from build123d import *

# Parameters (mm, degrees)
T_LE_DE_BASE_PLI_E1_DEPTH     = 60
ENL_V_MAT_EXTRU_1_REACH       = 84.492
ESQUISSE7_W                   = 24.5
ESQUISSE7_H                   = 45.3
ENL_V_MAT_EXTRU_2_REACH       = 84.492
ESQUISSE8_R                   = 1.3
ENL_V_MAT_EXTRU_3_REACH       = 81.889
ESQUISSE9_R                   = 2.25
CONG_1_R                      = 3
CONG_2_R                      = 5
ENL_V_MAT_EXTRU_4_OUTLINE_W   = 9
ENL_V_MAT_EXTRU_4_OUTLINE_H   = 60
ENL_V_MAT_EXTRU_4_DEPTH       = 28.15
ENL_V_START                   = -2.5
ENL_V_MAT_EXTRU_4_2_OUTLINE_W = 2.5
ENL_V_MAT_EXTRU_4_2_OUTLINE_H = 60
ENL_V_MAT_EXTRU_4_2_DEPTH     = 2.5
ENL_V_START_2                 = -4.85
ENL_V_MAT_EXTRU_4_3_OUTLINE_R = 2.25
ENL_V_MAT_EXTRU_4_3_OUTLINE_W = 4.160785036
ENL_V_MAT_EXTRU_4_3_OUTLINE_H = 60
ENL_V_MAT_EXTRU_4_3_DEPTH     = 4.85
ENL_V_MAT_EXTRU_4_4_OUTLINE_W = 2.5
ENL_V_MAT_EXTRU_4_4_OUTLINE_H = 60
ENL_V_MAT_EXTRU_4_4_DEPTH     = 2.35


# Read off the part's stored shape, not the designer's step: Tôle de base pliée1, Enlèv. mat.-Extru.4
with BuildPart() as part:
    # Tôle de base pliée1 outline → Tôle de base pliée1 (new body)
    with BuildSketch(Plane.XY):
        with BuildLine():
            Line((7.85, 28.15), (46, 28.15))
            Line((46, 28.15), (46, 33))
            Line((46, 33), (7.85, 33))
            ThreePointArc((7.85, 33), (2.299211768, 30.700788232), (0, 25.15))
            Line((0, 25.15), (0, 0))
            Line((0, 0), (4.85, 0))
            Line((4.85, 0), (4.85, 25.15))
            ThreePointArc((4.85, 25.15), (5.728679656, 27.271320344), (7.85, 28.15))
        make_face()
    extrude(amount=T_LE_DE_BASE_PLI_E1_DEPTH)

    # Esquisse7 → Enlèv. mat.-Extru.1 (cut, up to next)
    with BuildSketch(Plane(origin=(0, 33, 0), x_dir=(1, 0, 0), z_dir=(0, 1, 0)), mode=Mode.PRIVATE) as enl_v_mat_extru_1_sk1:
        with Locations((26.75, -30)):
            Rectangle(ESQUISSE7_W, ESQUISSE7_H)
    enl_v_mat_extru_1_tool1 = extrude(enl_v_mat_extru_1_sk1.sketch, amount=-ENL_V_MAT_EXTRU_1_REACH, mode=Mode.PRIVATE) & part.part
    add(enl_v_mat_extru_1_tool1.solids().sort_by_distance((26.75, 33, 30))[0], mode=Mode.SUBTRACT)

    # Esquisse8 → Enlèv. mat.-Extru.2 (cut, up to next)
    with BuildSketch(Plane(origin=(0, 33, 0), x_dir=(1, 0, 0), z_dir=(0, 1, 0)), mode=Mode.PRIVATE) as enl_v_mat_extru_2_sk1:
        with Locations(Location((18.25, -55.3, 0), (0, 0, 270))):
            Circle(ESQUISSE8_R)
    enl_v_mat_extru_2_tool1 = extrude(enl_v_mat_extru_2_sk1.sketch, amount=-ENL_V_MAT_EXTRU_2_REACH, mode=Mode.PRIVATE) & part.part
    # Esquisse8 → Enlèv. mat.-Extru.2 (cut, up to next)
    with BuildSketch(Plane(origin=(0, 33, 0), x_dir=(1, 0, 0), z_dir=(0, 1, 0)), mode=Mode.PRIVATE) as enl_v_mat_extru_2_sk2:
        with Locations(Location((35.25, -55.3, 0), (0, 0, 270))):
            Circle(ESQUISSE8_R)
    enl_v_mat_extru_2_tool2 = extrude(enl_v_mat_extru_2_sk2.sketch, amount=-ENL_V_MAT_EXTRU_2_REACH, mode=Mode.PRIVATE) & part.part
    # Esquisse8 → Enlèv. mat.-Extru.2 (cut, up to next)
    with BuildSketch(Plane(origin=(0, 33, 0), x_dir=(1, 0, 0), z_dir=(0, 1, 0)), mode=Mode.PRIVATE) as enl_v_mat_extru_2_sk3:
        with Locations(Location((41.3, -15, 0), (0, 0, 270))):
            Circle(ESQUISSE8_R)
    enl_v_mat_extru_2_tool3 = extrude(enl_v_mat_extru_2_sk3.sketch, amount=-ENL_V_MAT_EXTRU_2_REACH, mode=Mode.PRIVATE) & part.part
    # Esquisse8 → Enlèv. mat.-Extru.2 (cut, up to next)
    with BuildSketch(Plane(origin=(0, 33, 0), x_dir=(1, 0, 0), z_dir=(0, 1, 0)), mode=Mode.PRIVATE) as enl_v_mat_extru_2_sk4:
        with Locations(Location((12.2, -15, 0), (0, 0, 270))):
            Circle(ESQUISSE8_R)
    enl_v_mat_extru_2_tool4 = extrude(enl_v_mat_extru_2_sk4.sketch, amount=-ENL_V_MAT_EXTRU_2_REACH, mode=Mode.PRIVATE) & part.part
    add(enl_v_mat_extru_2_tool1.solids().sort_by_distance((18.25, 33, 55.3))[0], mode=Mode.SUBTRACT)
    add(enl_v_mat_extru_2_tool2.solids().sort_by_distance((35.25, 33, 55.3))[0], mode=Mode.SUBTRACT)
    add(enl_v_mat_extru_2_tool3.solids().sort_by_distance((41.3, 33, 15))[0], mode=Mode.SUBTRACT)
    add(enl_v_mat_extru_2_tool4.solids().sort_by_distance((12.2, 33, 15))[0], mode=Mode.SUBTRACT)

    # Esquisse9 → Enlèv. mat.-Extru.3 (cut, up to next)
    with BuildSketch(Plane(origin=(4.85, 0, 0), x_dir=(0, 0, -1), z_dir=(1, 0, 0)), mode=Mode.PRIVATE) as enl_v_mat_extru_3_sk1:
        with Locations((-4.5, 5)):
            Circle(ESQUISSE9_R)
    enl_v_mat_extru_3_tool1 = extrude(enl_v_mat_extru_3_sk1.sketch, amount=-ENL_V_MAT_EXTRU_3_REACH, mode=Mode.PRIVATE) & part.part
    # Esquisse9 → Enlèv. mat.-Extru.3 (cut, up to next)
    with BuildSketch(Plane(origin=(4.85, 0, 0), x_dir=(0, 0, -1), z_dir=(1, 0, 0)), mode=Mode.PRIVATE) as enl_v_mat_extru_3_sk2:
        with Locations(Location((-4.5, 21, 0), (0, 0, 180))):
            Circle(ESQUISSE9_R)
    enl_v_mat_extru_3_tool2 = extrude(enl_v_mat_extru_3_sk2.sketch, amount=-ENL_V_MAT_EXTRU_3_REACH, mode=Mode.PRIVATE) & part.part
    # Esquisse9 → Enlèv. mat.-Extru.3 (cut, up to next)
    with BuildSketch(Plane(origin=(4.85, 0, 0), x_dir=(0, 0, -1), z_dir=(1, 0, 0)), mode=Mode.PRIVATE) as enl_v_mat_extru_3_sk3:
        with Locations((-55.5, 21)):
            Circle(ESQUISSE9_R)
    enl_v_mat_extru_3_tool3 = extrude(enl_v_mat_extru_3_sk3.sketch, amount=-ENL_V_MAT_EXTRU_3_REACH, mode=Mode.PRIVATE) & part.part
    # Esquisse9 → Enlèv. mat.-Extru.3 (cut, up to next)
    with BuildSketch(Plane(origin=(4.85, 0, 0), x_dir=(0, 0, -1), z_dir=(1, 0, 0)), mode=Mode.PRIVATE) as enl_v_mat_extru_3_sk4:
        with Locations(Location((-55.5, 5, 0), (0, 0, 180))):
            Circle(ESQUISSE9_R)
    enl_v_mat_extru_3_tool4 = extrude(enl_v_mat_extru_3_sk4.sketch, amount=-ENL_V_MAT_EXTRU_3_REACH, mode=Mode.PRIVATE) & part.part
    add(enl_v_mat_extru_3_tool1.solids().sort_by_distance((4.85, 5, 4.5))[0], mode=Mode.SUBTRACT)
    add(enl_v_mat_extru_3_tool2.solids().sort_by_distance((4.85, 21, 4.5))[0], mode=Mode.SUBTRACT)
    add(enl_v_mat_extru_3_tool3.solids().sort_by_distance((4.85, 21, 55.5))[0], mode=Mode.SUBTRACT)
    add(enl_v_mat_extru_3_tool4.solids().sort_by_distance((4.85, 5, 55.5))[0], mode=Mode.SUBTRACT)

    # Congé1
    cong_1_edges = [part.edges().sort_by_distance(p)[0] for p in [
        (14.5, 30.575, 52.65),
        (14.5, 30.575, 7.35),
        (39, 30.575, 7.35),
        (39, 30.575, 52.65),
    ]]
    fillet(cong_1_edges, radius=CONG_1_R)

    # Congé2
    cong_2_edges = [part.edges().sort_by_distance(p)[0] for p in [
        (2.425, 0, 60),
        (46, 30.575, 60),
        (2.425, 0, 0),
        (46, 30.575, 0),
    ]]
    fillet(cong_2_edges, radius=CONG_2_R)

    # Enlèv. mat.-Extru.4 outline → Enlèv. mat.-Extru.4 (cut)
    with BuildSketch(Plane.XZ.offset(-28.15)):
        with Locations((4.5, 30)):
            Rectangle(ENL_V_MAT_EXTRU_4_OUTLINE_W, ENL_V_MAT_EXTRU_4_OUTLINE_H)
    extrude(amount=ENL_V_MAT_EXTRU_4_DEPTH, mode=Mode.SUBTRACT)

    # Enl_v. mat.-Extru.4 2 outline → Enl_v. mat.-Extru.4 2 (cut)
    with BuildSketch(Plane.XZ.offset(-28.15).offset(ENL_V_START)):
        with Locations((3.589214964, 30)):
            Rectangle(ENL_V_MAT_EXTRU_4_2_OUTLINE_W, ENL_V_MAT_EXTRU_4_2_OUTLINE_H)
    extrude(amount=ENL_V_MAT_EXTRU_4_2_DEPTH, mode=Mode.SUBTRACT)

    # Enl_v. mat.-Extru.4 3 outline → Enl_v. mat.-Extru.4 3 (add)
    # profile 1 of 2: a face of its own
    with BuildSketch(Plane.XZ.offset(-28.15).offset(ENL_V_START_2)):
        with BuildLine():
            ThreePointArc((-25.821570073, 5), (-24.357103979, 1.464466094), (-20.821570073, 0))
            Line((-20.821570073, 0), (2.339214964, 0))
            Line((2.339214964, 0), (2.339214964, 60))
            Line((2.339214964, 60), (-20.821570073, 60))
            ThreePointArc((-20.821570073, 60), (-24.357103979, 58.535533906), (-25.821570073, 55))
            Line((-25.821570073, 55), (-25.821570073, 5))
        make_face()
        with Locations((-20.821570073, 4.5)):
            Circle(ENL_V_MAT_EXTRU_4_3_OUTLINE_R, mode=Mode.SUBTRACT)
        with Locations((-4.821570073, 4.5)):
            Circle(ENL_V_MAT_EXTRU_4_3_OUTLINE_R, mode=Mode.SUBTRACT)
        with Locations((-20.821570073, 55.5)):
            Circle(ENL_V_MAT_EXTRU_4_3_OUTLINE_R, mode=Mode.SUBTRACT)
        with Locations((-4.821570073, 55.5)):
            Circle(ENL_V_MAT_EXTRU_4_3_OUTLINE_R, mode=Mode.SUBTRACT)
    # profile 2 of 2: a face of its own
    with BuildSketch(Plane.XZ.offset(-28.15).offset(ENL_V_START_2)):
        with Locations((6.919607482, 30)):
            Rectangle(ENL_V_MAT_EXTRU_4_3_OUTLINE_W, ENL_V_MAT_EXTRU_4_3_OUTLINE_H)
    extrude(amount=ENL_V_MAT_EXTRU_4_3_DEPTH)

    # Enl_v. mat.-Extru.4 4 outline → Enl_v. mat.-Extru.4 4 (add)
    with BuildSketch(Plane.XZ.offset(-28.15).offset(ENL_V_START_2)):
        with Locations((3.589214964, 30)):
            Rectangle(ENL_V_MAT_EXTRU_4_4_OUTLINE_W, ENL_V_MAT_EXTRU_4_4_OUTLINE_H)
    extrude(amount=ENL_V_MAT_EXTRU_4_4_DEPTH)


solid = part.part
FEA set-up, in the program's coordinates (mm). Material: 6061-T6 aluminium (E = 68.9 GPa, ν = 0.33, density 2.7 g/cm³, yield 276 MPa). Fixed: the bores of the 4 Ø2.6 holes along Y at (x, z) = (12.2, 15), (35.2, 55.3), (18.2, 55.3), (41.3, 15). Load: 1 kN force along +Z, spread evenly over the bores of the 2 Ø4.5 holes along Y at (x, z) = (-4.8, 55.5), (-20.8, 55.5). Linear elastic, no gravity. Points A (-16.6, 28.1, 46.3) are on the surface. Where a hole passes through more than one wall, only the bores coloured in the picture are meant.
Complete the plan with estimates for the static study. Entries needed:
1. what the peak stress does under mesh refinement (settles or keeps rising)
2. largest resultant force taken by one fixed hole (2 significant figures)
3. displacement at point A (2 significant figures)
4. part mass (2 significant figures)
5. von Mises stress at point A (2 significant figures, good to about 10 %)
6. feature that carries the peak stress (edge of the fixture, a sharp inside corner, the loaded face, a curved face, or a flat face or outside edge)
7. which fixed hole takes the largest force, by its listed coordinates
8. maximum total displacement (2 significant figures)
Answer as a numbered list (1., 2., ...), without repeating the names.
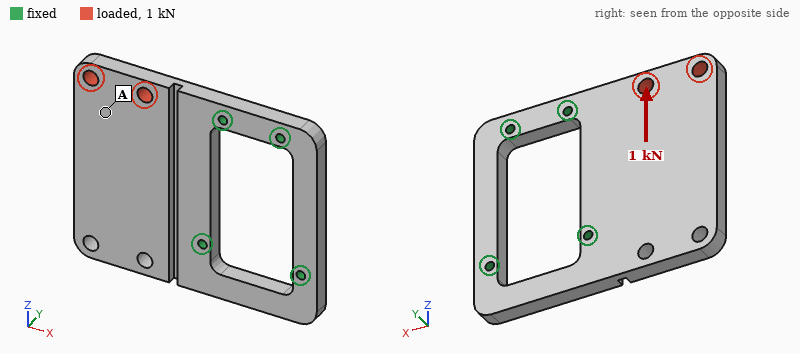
1. keeps rising
2. 890 N
3. 13 µm
4. 40 g
5. 6.6 MPa
6. edge of the fixture
7. (12.2, 15)
8. 18 µm
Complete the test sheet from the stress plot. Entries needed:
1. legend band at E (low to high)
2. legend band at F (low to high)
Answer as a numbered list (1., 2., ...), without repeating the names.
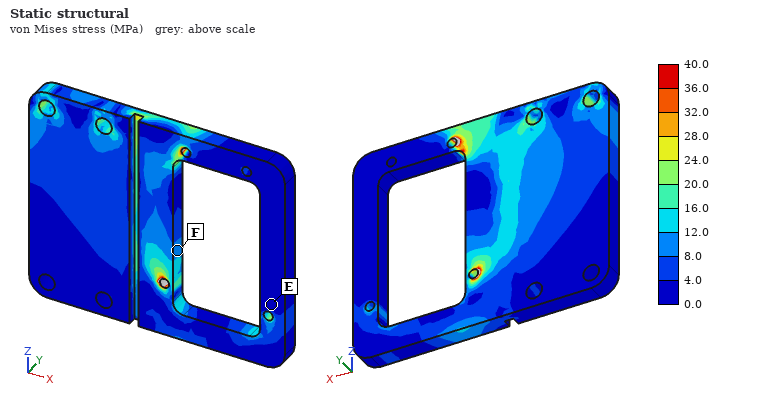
1. 0.0 to 4.0 MPa
2. 8.0 to 12.0 MPa
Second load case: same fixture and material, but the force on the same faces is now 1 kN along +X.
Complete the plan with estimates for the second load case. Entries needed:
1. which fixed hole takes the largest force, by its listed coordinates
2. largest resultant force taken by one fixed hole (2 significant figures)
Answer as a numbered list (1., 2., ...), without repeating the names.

1. (18.2, 55.3)
2. 960 N
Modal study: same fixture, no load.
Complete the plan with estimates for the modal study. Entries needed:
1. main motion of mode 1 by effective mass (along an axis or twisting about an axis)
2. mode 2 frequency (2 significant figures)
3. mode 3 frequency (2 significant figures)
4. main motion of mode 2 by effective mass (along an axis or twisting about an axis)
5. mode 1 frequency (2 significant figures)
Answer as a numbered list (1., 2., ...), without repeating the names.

1. along Y
2. 3700 Hz
3. 8700 Hz
4. twisting about X
5. 1400 Hz
